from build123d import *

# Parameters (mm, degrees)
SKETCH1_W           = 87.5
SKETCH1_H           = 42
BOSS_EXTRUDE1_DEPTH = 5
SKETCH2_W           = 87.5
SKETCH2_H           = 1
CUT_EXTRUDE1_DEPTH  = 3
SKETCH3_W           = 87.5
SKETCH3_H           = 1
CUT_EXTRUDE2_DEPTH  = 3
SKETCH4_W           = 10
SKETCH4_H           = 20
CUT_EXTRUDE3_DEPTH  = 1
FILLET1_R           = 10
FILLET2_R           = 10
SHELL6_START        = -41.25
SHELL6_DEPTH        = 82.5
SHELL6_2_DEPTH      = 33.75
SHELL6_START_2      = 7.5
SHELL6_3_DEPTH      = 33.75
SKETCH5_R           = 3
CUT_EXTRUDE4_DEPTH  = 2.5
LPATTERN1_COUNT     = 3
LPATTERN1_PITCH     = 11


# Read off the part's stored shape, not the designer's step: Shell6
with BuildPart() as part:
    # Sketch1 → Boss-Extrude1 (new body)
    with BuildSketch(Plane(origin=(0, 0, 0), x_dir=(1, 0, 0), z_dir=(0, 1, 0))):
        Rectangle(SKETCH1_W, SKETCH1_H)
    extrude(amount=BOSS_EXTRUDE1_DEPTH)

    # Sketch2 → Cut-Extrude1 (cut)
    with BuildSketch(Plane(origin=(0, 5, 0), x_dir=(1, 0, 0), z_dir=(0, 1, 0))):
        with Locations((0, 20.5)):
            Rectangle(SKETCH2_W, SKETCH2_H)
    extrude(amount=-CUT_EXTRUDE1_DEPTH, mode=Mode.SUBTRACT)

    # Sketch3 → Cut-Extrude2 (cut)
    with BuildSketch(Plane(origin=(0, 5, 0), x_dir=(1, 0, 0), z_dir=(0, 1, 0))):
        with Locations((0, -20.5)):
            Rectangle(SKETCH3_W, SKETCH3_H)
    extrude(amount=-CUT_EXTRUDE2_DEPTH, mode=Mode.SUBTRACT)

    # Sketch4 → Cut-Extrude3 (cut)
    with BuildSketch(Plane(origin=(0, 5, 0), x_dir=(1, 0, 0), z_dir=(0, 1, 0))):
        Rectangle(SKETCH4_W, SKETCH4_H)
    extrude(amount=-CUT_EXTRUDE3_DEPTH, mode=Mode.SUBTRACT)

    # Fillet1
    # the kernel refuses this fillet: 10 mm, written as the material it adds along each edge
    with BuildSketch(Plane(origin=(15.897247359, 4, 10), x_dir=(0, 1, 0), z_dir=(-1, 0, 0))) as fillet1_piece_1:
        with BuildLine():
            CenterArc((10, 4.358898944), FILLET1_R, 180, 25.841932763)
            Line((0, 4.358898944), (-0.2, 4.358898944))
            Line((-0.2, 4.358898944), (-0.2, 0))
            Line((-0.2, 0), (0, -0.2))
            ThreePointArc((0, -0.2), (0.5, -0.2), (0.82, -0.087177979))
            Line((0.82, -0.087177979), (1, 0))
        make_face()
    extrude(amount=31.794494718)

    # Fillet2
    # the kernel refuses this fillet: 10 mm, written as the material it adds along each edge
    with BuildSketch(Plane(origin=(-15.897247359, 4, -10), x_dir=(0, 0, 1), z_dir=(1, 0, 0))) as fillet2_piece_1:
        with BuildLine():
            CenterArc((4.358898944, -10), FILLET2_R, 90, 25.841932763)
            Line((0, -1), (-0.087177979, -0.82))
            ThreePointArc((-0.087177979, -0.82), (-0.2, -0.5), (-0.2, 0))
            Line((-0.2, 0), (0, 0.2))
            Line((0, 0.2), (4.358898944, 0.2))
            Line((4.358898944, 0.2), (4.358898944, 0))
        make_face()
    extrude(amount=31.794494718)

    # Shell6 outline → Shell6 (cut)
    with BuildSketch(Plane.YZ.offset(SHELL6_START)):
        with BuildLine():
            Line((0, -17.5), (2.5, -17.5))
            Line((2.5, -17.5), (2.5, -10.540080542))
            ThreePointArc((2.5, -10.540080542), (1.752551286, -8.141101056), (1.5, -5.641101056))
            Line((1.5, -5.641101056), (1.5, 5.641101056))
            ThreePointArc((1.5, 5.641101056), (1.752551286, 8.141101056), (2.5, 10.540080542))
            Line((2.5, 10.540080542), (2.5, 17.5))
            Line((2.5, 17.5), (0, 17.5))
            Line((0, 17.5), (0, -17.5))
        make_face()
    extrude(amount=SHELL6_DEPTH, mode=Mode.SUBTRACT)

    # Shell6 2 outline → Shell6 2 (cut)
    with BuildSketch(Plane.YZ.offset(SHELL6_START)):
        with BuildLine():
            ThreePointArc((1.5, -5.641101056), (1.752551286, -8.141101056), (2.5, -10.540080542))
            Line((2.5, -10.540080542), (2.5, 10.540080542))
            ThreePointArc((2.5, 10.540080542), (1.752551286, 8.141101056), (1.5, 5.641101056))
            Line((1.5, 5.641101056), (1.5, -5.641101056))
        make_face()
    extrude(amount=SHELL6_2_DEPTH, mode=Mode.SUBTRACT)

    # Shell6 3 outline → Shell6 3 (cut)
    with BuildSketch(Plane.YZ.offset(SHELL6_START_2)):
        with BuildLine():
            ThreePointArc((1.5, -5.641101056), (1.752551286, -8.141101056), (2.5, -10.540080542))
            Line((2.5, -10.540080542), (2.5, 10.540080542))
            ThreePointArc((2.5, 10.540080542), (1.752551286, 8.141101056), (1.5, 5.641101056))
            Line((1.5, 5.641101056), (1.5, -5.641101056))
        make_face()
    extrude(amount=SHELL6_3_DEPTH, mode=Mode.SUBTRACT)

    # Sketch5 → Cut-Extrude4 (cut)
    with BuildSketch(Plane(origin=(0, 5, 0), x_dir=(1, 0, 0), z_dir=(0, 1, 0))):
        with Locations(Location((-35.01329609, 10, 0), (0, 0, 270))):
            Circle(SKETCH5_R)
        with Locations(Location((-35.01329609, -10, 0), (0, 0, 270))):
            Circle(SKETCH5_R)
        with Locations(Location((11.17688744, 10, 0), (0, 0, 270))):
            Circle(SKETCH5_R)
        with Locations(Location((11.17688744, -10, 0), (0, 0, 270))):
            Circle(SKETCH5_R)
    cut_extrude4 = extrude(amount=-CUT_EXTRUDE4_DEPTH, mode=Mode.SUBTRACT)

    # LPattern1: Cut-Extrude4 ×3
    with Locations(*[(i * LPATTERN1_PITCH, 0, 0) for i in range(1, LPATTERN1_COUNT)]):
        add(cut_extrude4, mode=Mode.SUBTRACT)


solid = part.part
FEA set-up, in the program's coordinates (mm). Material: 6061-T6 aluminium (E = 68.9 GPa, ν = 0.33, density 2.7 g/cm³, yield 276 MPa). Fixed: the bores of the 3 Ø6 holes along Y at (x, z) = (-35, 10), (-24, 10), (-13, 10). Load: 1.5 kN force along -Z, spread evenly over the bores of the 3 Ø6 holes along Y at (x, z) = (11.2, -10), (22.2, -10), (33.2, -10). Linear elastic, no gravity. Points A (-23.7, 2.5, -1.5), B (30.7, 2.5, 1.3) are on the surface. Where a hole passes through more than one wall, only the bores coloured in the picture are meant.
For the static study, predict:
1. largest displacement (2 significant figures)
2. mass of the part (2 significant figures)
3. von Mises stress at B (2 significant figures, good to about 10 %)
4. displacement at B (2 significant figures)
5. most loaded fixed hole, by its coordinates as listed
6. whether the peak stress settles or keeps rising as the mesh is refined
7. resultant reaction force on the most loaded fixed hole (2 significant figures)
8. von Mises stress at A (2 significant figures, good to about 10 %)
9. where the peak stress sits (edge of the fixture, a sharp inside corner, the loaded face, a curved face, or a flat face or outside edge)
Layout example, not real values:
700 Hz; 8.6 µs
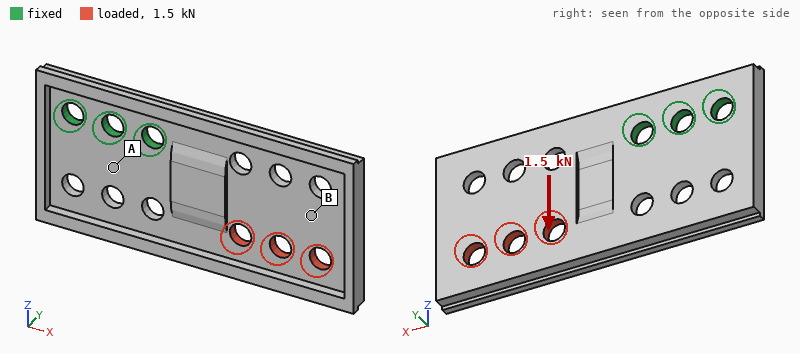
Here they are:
0.18 mm; 27 g; 15 MPa; 0.13 mm; (-13, 10); keeps rising; 3.2 kN; 60 MPa; edge of the fixture
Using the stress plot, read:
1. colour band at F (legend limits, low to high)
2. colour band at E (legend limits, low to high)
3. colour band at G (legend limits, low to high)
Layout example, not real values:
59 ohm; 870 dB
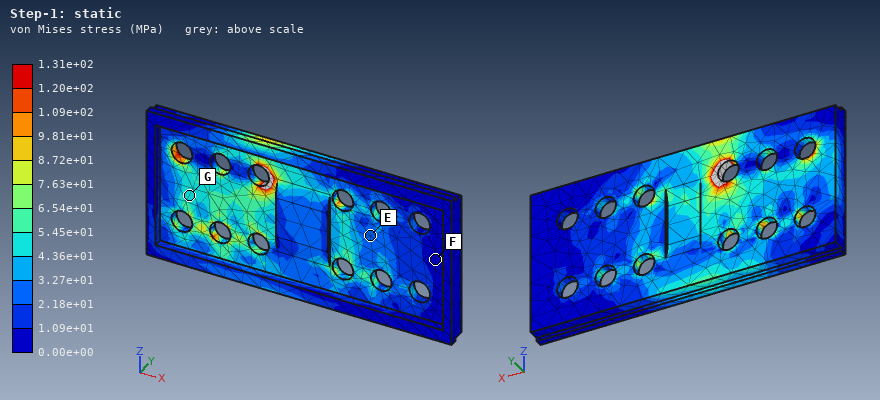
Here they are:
0.00e+00 to 1.09e+01 MPa; 2.18e+01 to 3.27e+01 MPa; 4.36e+01 to 5.45e+01 MPa
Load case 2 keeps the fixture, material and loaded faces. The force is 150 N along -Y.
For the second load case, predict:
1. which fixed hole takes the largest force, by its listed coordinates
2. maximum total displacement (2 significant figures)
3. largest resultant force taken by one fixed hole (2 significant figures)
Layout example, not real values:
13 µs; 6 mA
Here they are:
(-13, 10); 1.0 mm; 300 N
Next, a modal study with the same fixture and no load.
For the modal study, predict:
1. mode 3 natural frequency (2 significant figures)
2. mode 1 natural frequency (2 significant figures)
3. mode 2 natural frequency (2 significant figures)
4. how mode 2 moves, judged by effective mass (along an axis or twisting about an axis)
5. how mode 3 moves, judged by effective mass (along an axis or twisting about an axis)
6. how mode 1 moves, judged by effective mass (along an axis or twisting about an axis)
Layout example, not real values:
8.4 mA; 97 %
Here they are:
2900 Hz; 760 Hz; 1600 Hz; twisting about X; along Y; along Y
